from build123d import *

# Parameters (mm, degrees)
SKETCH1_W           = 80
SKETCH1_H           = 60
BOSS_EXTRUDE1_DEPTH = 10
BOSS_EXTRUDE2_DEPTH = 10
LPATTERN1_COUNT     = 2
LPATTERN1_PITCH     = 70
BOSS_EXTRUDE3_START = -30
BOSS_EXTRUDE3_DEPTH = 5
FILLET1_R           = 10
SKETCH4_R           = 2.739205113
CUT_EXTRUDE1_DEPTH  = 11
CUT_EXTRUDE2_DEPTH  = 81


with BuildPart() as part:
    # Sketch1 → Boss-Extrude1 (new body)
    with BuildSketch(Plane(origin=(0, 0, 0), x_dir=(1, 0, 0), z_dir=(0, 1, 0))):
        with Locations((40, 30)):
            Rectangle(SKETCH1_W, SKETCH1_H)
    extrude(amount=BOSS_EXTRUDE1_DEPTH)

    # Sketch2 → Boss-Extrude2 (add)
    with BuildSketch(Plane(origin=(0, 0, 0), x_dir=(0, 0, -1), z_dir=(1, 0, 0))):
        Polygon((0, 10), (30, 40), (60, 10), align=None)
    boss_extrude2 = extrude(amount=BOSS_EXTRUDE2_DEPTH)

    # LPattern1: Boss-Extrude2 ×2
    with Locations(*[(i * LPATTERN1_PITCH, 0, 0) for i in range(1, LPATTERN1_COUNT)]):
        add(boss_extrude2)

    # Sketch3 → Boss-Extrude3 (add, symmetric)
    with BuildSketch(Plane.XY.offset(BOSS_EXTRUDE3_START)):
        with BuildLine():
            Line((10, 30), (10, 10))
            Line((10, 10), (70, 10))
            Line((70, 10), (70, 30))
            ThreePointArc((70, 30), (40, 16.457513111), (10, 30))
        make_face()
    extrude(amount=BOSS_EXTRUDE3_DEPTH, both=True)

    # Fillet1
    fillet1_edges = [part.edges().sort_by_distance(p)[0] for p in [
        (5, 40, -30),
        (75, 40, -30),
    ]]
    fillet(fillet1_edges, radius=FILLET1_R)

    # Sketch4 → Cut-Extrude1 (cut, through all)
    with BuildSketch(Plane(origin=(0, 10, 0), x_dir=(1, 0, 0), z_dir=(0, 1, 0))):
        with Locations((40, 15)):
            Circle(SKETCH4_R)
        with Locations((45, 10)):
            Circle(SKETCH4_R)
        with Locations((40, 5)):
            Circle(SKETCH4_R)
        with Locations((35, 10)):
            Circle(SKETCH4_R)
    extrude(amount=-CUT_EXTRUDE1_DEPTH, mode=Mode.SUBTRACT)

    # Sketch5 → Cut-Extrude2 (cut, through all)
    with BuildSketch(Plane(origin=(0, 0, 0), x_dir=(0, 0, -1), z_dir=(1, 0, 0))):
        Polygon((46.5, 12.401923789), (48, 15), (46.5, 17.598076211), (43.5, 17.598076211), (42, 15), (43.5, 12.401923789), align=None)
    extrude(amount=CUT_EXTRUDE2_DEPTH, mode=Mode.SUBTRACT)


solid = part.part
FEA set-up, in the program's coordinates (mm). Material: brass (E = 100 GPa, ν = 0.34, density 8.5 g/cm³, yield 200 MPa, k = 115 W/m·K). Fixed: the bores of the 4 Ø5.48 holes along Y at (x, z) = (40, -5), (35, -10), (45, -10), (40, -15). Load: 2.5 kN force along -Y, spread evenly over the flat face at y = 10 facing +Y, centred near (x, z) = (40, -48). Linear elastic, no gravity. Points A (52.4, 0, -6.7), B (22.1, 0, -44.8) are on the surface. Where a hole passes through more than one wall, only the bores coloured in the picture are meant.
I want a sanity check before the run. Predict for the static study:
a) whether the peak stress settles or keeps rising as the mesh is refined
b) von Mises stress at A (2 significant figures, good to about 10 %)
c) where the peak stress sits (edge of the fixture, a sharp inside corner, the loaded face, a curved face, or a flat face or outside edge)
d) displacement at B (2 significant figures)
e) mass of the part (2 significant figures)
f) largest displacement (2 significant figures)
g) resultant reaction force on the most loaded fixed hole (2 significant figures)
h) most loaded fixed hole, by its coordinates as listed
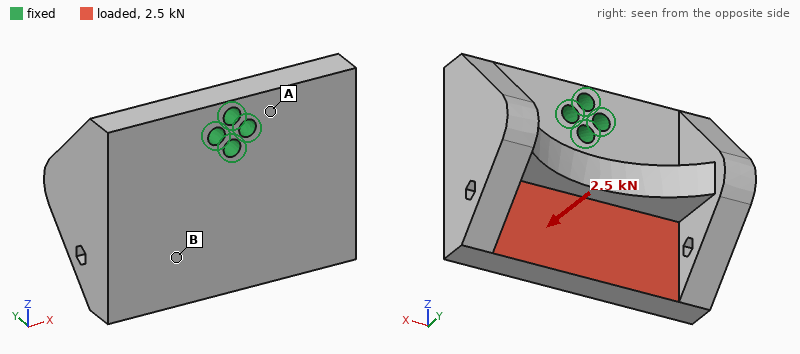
keeps rising
43 MPa
edge of the fixture
62 µm
600 g
97 µm
3.7 kN
(40, -15)
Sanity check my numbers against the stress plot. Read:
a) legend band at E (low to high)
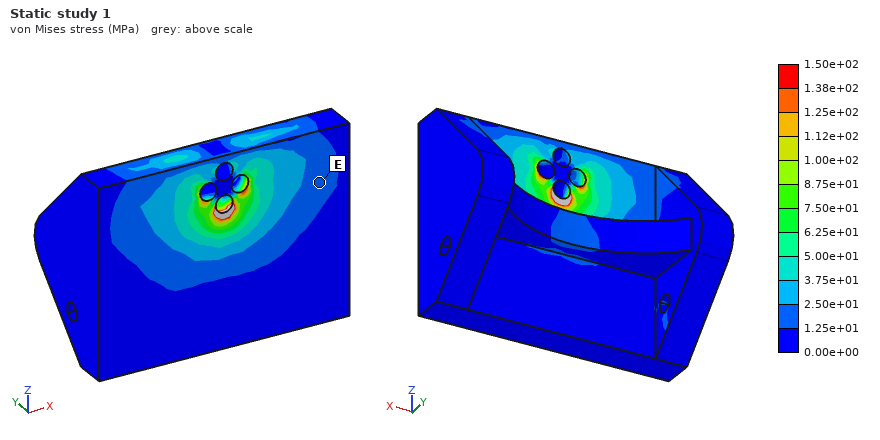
1.25e+01 to 2.50e+01 MPa
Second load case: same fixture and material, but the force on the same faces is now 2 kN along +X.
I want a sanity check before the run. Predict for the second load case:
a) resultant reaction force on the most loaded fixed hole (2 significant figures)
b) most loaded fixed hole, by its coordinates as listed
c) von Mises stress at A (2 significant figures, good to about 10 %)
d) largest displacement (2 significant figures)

3.8 kN
(40, -15)
18 MPa
29 µm
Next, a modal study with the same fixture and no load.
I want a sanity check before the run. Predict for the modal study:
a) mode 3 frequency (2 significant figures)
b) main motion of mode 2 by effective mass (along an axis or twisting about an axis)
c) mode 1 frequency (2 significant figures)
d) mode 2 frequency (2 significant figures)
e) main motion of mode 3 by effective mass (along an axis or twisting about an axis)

2400 Hz
along Y
1700 Hz
1700 Hz
along X
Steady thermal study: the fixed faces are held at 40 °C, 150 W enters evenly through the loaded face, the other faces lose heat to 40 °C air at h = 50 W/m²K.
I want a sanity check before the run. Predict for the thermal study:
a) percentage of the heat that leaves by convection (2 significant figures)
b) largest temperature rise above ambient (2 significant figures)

18 %
65 K
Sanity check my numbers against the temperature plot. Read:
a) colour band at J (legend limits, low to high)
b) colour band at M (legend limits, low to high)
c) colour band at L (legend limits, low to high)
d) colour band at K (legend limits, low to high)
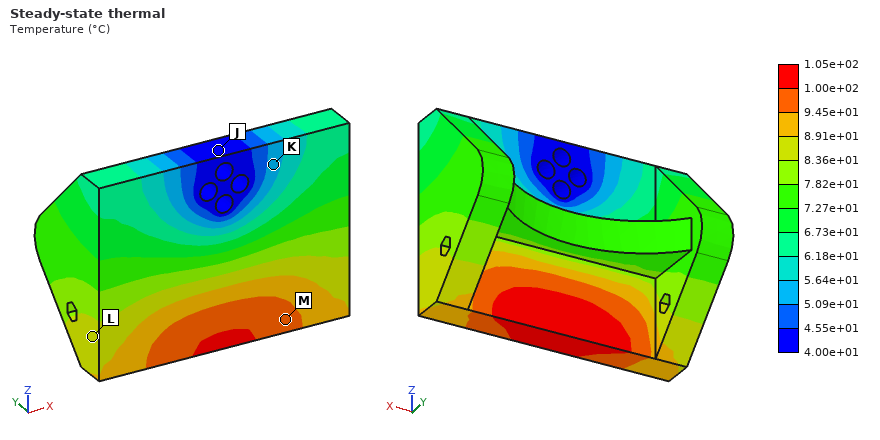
4.00e+01 to 4.55e+01 °C
9.45e+01 to 1.00e+02 °C
8.36e+01 to 8.91e+01 °C
5.09e+01 to 5.64e+01 °C
